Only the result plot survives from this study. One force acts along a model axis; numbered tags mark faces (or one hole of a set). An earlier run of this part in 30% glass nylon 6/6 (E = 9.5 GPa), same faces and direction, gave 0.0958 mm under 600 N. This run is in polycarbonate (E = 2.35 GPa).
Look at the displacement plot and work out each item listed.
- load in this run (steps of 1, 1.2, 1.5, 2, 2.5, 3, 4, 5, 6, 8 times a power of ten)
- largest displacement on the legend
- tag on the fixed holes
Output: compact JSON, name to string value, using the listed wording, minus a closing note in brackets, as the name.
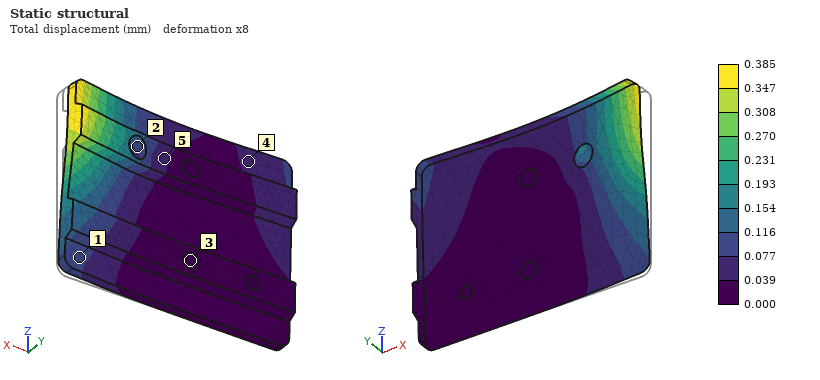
{"load in this run": "600 N", "largest displacement on the legend": "0.385 mm", "tag on the fixed holes": "3"}
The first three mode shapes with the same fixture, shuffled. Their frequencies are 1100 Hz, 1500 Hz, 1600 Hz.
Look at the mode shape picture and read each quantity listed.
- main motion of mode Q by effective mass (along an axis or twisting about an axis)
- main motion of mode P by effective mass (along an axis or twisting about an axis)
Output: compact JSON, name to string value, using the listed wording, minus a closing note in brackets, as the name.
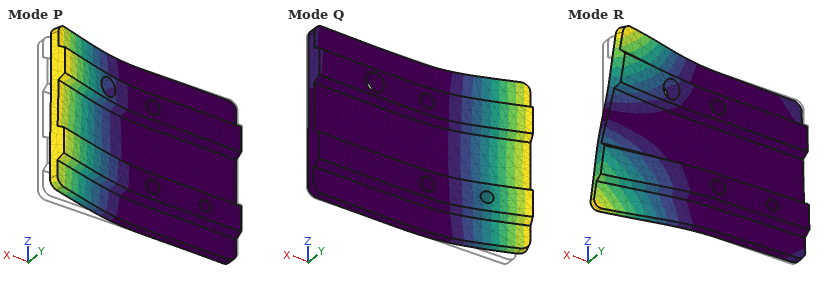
{"main motion of mode Q by effective mass": "along Y", "main motion of mode P by effective mass": "along Y"}
